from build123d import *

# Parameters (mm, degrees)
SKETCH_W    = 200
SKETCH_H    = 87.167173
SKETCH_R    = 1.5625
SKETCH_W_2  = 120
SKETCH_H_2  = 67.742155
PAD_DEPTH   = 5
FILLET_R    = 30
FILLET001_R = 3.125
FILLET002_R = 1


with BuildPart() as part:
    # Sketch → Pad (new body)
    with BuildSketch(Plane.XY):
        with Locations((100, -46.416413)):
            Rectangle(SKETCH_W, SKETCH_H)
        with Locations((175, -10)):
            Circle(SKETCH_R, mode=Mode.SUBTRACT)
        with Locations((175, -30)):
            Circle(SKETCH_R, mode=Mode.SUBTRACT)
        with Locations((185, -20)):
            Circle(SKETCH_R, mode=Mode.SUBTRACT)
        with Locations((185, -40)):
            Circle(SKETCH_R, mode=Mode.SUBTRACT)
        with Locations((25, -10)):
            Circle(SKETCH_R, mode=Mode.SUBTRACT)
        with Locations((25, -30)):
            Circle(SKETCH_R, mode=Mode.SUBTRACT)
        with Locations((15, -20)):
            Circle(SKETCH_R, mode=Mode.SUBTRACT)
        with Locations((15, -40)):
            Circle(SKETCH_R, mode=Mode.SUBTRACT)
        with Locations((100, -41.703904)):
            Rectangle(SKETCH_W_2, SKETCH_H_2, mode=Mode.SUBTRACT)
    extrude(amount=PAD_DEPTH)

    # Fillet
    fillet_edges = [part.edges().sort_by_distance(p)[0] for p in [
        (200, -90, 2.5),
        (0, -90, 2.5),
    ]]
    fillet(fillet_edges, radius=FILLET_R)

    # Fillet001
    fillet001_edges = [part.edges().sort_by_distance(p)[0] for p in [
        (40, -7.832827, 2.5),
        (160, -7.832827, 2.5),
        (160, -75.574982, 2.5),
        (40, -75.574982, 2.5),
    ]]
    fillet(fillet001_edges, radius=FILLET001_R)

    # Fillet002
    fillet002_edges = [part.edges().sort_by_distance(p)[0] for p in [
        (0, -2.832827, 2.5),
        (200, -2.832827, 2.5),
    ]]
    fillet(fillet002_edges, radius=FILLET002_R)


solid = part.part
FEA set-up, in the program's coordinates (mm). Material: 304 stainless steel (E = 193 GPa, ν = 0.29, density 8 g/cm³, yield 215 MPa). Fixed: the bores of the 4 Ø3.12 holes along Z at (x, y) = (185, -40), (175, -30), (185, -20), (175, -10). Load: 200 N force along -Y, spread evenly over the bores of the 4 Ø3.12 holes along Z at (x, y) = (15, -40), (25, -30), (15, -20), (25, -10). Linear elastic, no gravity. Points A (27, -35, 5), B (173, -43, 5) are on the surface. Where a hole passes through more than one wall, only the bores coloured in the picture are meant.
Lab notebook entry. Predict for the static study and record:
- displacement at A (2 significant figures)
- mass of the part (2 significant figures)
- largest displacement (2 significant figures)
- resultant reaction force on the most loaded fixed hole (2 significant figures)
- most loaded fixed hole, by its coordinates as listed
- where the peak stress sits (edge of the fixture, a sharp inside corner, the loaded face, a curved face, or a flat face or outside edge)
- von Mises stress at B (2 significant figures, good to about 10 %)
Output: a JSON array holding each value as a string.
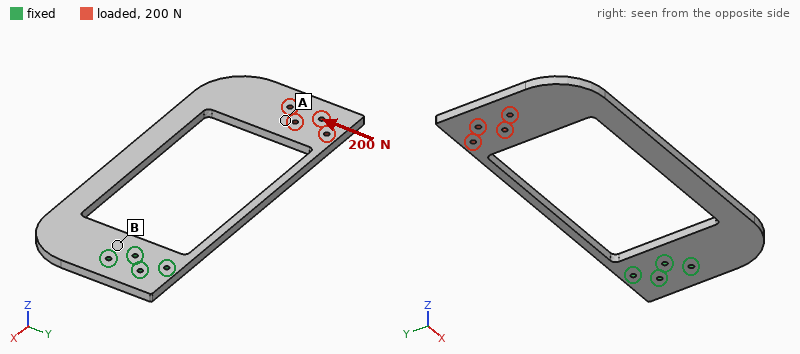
["0.20 mm", "350 g", "0.21 mm", "880 N", "(185, -40)", "a curved face", "11 MPa"]
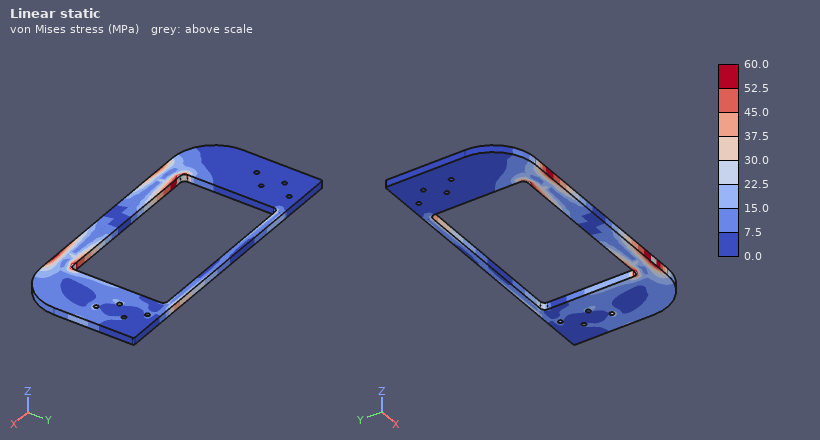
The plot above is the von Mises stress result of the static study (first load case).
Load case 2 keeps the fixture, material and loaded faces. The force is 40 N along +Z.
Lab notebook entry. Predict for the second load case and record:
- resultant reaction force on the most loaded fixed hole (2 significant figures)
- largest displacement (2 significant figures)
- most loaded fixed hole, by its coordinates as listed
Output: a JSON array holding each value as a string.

["190 N", "1.6 mm", "(175, -30)"]
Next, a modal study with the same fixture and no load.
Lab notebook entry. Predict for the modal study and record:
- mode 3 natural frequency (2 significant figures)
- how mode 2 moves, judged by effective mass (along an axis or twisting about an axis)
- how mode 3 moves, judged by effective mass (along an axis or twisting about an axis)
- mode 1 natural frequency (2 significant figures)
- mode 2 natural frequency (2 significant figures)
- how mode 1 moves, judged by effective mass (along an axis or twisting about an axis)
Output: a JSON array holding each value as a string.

["390 Hz", "twisting about X", "along Y", "73 Hz", "290 Hz", "along Z"]
